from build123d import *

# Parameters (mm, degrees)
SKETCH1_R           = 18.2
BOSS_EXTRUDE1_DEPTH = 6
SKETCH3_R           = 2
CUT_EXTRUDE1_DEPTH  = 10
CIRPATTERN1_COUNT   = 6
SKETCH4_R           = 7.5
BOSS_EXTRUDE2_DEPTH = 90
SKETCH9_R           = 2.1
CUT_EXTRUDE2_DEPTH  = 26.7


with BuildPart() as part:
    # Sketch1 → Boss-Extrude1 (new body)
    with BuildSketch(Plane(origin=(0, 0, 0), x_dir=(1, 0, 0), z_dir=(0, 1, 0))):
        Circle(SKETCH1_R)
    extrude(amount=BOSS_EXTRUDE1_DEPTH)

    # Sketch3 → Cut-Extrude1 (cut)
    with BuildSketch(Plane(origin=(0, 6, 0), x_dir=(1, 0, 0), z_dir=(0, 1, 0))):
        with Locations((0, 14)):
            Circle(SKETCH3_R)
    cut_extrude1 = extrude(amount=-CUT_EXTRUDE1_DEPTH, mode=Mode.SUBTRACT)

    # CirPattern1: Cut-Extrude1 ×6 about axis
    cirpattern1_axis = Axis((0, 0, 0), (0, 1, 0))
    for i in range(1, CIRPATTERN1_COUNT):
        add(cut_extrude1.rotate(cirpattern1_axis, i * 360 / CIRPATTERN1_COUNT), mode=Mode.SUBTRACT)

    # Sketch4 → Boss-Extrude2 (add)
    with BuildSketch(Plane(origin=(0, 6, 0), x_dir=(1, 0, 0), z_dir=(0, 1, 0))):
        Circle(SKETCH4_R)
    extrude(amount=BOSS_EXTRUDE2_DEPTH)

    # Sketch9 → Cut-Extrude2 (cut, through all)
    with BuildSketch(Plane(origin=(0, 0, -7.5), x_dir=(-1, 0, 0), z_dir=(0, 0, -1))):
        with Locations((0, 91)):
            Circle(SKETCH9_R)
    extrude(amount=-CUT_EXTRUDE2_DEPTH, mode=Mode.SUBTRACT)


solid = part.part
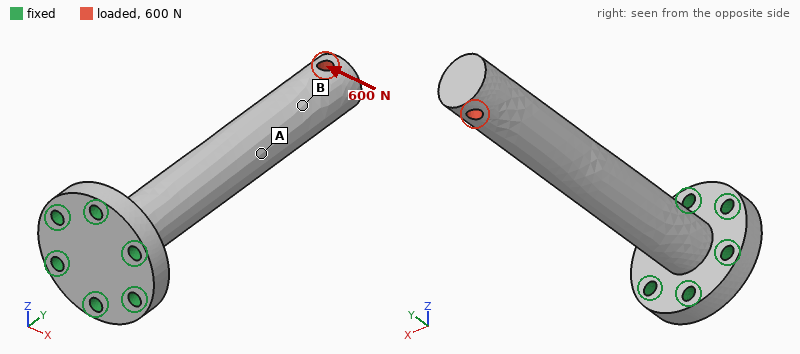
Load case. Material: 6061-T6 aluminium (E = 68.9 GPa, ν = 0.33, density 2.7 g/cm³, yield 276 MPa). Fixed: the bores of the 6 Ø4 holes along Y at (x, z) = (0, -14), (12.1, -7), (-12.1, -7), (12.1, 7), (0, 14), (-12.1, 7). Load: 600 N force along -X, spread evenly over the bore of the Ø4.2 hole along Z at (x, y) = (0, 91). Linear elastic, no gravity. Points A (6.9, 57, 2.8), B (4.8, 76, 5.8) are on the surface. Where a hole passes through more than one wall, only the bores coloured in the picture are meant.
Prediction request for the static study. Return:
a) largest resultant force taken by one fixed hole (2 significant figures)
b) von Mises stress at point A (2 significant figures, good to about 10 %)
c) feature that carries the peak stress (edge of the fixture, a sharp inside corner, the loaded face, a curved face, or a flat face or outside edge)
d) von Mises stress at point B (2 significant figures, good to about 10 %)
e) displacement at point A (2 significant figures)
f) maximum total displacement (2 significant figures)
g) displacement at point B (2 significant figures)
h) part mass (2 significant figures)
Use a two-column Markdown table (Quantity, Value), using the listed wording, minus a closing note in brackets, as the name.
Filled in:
| Quantity | Value |
|---|---|
| largest resultant force taken by one fixed hole | 1.3 kN |
| von Mises stress at point A | 57 MPa |
| feature that carries the peak stress | a curved face |
| von Mises stress at point B | 19 MPa |
| displacement at point A | 0.41 mm |
| maximum total displacement | 0.94 mm |
| displacement at point B | 0.65 mm |
| part mass | 58 g |
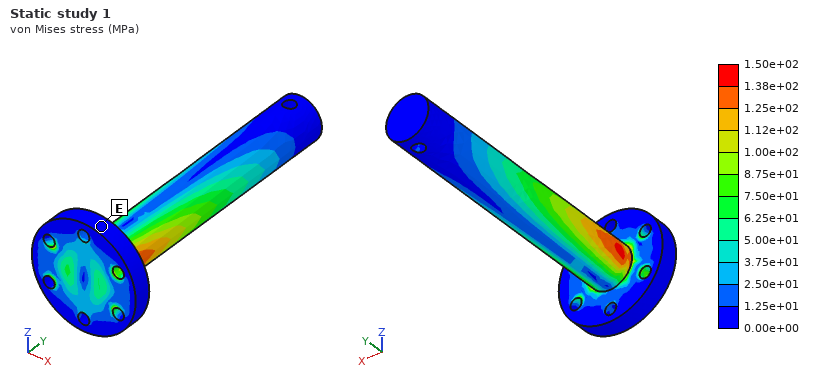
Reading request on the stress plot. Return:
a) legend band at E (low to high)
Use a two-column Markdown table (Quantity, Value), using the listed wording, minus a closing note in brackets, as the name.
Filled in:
| Quantity | Value |
|---|---|
| legend band at E | 0.00e+00 to 1.25e+01 MPa |
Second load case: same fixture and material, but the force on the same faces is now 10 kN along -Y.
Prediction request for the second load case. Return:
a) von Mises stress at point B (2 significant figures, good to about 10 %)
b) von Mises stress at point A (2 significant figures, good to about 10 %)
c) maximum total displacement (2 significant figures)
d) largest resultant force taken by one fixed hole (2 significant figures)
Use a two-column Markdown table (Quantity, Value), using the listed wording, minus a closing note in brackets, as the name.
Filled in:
| Quantity | Value |
|---|---|
| von Mises stress at point B | 57 MPa |
| von Mises stress at point A | 56 MPa |
| maximum total displacement | 93 µm |
| largest resultant force taken by one fixed hole | 1.8 kN |
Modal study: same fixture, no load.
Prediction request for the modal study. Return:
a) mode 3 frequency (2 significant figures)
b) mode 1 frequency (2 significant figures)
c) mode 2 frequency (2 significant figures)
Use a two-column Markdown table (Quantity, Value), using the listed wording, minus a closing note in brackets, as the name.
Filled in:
| Quantity | Value |
|---|---|
| mode 3 frequency | 6900 Hz |
| mode 1 frequency | 1200 Hz |
| mode 2 frequency | 1200 Hz |
